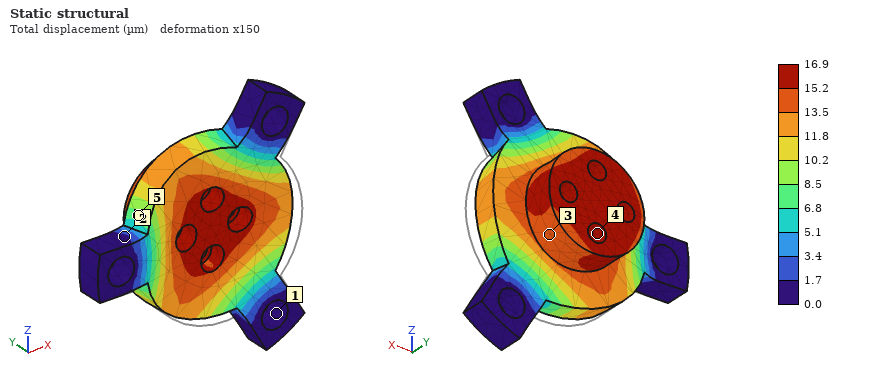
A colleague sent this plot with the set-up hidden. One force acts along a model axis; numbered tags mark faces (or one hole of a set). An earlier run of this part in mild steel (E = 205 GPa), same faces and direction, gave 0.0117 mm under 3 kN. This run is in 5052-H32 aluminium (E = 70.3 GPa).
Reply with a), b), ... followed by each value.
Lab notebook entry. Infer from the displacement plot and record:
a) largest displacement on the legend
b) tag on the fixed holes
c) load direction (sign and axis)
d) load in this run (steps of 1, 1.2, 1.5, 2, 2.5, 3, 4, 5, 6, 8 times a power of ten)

a) 16.9 µm
b) 1
c) +Y
d) 1.5 kN
